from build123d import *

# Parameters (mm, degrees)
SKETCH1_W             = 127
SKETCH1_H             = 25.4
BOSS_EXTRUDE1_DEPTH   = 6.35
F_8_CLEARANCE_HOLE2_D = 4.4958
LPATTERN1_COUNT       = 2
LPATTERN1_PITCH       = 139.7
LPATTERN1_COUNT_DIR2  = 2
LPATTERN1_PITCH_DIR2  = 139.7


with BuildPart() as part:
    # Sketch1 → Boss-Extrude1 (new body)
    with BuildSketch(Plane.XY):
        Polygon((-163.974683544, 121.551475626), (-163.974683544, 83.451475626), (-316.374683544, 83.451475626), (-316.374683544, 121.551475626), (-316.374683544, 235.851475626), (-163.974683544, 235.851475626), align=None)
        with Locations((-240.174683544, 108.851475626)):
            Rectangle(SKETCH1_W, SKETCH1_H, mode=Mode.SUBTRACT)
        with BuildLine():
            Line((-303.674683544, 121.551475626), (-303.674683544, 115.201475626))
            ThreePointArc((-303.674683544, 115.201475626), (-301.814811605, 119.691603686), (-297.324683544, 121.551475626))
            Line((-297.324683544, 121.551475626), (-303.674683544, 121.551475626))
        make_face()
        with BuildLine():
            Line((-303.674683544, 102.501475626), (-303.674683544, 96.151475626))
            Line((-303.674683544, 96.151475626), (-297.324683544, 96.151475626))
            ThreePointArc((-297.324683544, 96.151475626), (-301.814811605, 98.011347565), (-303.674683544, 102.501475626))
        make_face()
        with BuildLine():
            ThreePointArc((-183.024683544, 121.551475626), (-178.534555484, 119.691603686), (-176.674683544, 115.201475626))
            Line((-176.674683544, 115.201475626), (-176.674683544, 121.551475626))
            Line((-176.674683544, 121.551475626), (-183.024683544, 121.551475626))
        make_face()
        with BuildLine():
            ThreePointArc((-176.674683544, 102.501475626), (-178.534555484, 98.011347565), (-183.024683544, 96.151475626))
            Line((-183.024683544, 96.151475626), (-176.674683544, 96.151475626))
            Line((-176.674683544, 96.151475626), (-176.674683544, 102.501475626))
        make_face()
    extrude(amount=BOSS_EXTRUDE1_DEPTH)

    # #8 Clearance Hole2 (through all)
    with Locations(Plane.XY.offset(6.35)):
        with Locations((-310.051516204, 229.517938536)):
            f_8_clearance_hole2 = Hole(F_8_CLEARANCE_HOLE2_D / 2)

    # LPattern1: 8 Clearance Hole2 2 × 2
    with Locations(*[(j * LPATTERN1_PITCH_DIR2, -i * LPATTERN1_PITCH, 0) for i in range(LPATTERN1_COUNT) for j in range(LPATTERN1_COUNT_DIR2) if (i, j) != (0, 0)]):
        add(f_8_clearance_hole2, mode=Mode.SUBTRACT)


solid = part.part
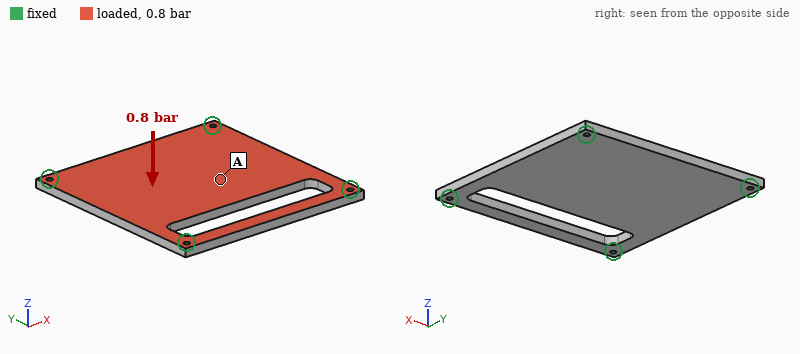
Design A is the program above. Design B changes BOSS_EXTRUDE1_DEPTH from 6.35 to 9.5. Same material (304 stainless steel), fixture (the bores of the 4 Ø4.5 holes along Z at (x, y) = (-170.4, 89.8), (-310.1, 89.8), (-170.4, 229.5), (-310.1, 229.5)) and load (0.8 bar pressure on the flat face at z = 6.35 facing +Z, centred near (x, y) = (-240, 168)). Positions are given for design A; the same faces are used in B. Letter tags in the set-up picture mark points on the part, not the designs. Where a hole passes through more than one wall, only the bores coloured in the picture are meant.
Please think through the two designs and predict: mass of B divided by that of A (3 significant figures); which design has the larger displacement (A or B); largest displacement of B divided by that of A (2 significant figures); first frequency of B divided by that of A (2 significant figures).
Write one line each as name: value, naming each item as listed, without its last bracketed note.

mass of B divided by that of A: 1.50
which design has the larger displacement: A
largest displacement of B divided by that of A: 0.33
first frequency of B divided by that of A: 1.4
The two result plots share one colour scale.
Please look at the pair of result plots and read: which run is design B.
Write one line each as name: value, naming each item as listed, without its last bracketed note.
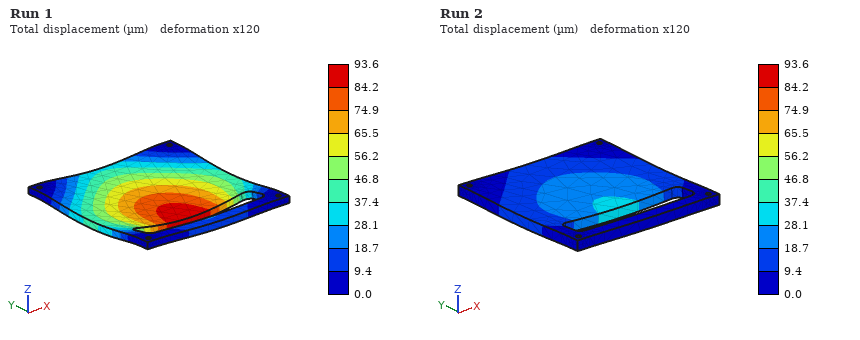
which run is design B: Run 2
